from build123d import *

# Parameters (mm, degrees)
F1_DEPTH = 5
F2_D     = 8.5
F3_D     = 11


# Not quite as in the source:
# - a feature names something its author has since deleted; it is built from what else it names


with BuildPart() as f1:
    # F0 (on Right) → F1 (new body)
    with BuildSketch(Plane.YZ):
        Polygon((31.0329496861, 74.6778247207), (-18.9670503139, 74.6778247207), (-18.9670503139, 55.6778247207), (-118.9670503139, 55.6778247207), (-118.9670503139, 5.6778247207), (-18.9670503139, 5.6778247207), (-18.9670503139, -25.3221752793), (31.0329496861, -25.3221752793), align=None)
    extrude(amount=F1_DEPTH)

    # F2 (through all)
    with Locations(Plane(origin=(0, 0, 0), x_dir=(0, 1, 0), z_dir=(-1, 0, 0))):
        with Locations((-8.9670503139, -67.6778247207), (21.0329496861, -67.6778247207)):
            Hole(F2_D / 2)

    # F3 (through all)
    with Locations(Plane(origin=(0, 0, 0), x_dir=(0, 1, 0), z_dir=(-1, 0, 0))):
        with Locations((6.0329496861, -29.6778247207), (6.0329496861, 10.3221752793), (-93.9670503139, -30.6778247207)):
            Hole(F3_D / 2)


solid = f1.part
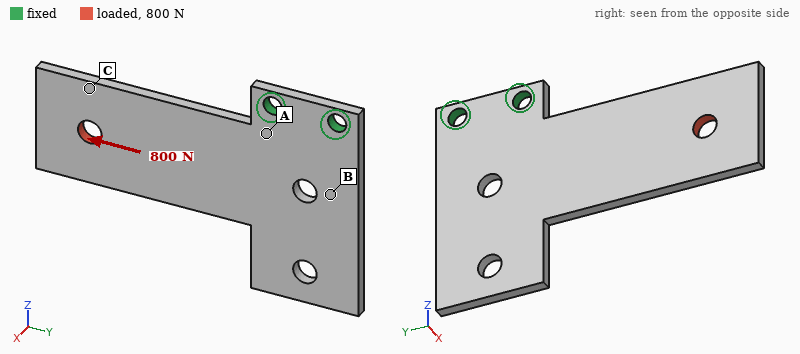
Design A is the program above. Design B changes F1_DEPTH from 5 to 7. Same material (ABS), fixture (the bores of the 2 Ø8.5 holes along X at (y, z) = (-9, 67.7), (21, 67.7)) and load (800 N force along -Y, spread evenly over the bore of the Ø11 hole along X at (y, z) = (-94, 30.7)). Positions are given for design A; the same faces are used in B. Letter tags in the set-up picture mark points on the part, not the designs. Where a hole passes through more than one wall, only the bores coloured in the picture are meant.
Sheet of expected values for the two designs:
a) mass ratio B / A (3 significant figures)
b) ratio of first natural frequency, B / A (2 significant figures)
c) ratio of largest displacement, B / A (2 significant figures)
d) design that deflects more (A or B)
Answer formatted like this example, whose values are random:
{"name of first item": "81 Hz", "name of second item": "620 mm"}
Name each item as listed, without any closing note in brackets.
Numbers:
{"mass ratio B / A": "1.40", "ratio of first natural frequency, B / A": "1.4", "ratio of largest displacement, B / A": "0.71", "design that deflects more": "A"}
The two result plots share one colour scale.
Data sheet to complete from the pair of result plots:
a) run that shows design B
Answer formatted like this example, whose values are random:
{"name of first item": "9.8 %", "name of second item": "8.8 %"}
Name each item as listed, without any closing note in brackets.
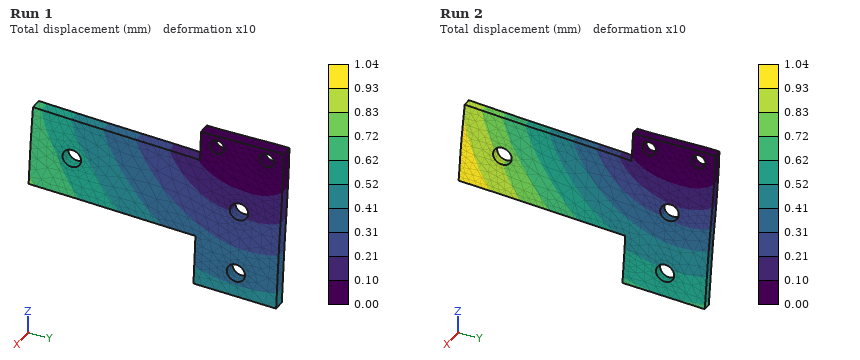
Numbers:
{"run that shows design B": "Run 1"}
